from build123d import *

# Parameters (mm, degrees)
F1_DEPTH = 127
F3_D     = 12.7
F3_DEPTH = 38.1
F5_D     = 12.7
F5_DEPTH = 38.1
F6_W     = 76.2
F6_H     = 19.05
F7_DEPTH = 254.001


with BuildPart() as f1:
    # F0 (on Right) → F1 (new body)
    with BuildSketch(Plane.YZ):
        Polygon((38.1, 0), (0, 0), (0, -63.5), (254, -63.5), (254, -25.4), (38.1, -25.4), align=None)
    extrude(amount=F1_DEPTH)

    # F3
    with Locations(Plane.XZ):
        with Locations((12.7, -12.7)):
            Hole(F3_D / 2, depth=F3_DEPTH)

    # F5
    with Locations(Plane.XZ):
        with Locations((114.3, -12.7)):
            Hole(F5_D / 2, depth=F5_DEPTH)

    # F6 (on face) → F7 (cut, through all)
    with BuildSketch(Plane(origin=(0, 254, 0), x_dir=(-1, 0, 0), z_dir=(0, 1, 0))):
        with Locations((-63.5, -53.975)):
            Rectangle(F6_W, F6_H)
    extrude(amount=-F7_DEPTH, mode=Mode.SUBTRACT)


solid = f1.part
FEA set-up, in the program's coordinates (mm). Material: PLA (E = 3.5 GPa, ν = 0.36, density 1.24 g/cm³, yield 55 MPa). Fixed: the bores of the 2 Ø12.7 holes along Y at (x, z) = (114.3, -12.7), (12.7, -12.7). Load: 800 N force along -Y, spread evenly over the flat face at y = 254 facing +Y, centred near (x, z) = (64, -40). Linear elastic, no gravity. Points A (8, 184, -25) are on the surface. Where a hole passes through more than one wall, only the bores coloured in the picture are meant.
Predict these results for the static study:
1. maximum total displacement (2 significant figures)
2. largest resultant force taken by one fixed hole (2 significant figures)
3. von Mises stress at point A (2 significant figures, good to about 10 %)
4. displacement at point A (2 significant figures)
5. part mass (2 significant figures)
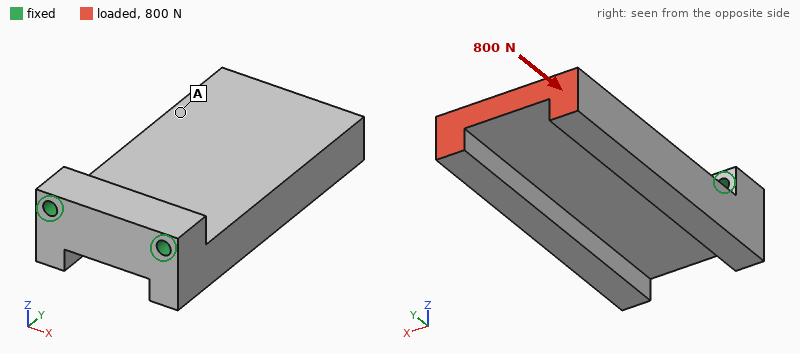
91 µm
400 N
0.24 MPa
60 µm
1.2 kg
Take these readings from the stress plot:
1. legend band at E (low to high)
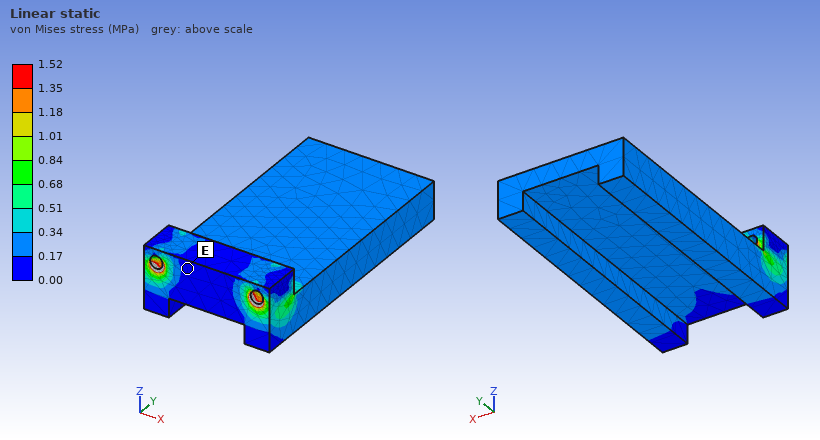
0.00 to 0.17 MPa
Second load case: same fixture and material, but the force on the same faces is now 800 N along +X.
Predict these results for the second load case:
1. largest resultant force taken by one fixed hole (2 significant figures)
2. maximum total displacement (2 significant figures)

1.8 kN
0.45 mm
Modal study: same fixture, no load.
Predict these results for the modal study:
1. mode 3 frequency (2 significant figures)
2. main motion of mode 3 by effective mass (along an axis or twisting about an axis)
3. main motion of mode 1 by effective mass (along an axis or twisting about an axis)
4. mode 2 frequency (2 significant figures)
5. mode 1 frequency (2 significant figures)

410 Hz
along X
along Z
370 Hz
150 Hz
